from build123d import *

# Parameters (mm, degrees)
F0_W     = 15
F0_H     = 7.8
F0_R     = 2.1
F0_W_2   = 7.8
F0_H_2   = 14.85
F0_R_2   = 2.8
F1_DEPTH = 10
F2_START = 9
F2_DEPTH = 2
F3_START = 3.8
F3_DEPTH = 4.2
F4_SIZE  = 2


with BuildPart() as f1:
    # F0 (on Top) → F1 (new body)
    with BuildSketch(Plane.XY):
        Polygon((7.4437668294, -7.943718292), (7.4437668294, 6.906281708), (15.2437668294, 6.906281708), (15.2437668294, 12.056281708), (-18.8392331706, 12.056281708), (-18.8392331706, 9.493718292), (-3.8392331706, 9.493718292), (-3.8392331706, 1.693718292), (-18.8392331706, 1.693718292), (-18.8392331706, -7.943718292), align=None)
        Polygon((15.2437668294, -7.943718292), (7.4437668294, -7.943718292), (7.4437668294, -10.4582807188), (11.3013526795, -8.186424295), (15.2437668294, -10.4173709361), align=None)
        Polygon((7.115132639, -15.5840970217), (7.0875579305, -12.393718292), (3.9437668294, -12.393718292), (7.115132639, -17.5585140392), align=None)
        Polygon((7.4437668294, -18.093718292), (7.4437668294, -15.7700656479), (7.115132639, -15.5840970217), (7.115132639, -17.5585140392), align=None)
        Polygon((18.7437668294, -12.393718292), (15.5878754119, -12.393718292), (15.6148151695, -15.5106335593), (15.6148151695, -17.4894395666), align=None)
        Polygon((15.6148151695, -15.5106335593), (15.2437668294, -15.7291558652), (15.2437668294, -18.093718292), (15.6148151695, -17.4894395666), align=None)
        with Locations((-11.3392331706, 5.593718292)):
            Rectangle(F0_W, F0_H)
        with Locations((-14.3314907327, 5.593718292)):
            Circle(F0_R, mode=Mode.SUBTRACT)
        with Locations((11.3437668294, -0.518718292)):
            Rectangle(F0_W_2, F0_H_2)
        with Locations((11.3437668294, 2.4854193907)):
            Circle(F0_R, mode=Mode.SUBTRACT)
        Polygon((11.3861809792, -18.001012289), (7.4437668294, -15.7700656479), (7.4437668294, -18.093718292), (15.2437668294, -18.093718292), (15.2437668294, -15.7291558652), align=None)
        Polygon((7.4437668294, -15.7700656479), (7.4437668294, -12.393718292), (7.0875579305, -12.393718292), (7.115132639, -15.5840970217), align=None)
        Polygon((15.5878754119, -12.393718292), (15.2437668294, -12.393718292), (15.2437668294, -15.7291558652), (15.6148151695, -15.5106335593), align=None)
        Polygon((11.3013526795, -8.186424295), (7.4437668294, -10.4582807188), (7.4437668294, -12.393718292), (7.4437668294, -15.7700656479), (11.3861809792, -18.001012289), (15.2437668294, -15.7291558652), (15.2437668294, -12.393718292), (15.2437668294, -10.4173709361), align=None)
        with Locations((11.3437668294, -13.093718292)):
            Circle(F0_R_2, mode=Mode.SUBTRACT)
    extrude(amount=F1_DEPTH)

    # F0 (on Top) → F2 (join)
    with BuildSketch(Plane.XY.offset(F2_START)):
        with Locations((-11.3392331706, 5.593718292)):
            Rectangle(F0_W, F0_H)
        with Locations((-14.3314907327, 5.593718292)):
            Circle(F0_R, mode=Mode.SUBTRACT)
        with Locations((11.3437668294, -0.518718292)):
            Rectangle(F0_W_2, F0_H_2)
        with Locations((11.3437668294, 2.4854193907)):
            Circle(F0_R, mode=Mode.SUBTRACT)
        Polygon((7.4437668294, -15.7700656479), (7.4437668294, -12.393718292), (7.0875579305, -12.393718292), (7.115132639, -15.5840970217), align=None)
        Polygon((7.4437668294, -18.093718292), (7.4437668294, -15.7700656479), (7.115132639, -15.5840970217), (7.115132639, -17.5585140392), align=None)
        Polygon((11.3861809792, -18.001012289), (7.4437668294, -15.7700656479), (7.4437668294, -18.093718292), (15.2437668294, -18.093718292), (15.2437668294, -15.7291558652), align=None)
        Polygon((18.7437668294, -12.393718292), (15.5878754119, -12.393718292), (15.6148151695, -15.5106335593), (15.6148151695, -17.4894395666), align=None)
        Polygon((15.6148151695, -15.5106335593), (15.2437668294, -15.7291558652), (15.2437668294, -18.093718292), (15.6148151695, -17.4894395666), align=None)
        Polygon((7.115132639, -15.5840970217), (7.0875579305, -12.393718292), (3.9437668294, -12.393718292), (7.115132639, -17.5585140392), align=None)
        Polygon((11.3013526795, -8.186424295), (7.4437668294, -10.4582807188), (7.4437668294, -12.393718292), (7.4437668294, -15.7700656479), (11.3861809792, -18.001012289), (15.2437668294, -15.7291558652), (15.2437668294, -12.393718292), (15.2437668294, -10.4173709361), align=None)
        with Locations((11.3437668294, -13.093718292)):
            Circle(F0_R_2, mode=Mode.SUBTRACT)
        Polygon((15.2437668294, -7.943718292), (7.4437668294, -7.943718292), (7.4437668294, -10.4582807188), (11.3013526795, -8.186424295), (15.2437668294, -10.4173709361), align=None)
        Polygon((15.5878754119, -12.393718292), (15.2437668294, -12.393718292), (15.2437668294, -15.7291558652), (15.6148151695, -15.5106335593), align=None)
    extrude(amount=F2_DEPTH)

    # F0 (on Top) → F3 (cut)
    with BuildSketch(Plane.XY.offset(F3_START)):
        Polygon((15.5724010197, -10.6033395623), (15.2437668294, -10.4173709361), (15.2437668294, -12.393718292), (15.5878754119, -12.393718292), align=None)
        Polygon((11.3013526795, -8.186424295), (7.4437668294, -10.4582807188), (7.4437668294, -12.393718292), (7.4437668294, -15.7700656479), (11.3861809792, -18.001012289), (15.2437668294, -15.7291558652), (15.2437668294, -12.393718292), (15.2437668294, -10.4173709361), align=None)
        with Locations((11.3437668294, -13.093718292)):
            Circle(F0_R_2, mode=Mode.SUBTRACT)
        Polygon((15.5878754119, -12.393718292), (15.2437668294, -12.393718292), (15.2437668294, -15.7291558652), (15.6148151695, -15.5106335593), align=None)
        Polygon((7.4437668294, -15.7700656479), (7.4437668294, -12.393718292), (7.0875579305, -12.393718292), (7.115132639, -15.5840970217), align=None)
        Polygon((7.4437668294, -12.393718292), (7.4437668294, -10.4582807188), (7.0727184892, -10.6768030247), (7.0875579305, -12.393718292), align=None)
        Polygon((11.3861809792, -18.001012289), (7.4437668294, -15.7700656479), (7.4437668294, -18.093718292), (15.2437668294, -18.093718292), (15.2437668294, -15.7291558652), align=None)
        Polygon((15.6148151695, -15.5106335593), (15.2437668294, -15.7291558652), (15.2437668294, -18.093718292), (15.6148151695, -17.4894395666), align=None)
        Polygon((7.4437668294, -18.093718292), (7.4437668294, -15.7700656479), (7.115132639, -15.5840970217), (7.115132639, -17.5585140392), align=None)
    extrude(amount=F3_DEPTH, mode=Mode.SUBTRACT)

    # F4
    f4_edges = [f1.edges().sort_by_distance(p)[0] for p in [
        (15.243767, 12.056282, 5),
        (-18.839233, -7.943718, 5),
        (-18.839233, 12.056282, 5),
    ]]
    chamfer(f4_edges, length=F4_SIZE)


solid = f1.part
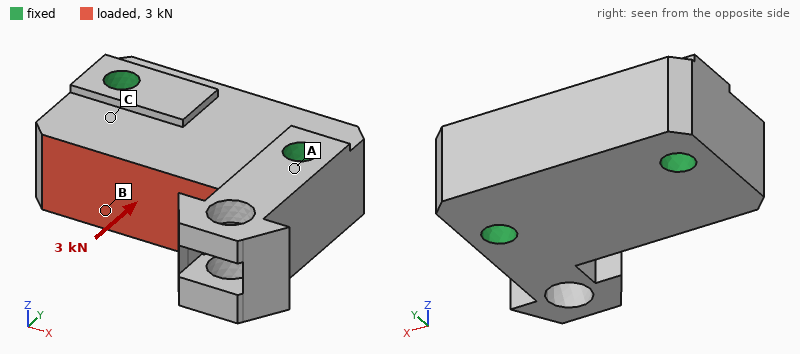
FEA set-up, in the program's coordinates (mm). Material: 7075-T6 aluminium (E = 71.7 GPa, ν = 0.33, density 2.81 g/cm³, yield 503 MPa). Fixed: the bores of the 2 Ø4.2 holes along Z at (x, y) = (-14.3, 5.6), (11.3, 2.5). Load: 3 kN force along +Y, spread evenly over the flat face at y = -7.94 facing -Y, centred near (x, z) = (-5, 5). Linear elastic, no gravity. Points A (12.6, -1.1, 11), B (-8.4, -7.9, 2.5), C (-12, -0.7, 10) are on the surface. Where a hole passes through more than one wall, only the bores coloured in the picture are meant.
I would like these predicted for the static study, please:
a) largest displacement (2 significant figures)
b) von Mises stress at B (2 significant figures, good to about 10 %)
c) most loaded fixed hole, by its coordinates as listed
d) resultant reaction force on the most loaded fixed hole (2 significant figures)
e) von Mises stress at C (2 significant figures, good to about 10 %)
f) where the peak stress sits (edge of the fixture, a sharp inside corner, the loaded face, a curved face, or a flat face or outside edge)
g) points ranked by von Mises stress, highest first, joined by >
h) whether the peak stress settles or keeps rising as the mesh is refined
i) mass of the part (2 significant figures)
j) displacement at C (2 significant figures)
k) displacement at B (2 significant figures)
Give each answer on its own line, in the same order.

4.0 µm
11 MPa
(-14.3, 5.6)
1.9 kN
18 MPa
edge of the fixture
C > B > A
keeps rising
21 g
1.4 µm
3.4 µm
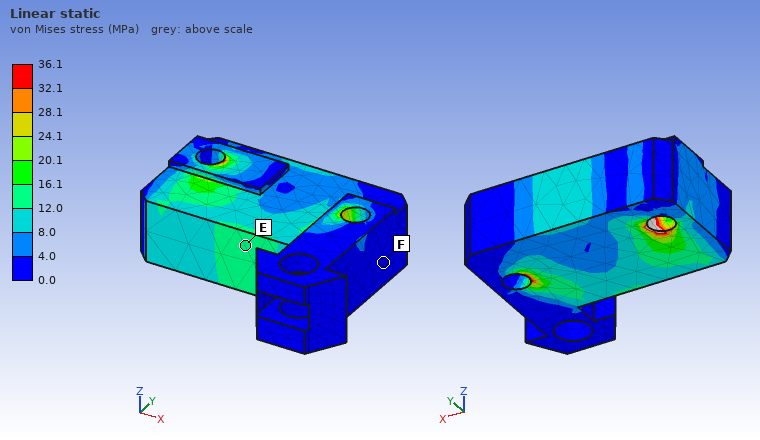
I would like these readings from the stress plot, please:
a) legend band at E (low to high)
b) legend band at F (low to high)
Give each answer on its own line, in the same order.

12.0 to 16.1 MPa
0.0 to 4.0 MPa
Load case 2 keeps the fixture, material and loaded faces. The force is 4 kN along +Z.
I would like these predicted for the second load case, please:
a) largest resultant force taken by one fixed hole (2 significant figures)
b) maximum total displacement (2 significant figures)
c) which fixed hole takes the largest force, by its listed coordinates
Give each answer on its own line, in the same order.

2.3 kN
34 µm
(-14.3, 5.6)
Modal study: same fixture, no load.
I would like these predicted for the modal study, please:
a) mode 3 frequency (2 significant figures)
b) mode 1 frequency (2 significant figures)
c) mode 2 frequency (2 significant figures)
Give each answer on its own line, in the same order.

29 kHz
18 kHz
20 kHz
